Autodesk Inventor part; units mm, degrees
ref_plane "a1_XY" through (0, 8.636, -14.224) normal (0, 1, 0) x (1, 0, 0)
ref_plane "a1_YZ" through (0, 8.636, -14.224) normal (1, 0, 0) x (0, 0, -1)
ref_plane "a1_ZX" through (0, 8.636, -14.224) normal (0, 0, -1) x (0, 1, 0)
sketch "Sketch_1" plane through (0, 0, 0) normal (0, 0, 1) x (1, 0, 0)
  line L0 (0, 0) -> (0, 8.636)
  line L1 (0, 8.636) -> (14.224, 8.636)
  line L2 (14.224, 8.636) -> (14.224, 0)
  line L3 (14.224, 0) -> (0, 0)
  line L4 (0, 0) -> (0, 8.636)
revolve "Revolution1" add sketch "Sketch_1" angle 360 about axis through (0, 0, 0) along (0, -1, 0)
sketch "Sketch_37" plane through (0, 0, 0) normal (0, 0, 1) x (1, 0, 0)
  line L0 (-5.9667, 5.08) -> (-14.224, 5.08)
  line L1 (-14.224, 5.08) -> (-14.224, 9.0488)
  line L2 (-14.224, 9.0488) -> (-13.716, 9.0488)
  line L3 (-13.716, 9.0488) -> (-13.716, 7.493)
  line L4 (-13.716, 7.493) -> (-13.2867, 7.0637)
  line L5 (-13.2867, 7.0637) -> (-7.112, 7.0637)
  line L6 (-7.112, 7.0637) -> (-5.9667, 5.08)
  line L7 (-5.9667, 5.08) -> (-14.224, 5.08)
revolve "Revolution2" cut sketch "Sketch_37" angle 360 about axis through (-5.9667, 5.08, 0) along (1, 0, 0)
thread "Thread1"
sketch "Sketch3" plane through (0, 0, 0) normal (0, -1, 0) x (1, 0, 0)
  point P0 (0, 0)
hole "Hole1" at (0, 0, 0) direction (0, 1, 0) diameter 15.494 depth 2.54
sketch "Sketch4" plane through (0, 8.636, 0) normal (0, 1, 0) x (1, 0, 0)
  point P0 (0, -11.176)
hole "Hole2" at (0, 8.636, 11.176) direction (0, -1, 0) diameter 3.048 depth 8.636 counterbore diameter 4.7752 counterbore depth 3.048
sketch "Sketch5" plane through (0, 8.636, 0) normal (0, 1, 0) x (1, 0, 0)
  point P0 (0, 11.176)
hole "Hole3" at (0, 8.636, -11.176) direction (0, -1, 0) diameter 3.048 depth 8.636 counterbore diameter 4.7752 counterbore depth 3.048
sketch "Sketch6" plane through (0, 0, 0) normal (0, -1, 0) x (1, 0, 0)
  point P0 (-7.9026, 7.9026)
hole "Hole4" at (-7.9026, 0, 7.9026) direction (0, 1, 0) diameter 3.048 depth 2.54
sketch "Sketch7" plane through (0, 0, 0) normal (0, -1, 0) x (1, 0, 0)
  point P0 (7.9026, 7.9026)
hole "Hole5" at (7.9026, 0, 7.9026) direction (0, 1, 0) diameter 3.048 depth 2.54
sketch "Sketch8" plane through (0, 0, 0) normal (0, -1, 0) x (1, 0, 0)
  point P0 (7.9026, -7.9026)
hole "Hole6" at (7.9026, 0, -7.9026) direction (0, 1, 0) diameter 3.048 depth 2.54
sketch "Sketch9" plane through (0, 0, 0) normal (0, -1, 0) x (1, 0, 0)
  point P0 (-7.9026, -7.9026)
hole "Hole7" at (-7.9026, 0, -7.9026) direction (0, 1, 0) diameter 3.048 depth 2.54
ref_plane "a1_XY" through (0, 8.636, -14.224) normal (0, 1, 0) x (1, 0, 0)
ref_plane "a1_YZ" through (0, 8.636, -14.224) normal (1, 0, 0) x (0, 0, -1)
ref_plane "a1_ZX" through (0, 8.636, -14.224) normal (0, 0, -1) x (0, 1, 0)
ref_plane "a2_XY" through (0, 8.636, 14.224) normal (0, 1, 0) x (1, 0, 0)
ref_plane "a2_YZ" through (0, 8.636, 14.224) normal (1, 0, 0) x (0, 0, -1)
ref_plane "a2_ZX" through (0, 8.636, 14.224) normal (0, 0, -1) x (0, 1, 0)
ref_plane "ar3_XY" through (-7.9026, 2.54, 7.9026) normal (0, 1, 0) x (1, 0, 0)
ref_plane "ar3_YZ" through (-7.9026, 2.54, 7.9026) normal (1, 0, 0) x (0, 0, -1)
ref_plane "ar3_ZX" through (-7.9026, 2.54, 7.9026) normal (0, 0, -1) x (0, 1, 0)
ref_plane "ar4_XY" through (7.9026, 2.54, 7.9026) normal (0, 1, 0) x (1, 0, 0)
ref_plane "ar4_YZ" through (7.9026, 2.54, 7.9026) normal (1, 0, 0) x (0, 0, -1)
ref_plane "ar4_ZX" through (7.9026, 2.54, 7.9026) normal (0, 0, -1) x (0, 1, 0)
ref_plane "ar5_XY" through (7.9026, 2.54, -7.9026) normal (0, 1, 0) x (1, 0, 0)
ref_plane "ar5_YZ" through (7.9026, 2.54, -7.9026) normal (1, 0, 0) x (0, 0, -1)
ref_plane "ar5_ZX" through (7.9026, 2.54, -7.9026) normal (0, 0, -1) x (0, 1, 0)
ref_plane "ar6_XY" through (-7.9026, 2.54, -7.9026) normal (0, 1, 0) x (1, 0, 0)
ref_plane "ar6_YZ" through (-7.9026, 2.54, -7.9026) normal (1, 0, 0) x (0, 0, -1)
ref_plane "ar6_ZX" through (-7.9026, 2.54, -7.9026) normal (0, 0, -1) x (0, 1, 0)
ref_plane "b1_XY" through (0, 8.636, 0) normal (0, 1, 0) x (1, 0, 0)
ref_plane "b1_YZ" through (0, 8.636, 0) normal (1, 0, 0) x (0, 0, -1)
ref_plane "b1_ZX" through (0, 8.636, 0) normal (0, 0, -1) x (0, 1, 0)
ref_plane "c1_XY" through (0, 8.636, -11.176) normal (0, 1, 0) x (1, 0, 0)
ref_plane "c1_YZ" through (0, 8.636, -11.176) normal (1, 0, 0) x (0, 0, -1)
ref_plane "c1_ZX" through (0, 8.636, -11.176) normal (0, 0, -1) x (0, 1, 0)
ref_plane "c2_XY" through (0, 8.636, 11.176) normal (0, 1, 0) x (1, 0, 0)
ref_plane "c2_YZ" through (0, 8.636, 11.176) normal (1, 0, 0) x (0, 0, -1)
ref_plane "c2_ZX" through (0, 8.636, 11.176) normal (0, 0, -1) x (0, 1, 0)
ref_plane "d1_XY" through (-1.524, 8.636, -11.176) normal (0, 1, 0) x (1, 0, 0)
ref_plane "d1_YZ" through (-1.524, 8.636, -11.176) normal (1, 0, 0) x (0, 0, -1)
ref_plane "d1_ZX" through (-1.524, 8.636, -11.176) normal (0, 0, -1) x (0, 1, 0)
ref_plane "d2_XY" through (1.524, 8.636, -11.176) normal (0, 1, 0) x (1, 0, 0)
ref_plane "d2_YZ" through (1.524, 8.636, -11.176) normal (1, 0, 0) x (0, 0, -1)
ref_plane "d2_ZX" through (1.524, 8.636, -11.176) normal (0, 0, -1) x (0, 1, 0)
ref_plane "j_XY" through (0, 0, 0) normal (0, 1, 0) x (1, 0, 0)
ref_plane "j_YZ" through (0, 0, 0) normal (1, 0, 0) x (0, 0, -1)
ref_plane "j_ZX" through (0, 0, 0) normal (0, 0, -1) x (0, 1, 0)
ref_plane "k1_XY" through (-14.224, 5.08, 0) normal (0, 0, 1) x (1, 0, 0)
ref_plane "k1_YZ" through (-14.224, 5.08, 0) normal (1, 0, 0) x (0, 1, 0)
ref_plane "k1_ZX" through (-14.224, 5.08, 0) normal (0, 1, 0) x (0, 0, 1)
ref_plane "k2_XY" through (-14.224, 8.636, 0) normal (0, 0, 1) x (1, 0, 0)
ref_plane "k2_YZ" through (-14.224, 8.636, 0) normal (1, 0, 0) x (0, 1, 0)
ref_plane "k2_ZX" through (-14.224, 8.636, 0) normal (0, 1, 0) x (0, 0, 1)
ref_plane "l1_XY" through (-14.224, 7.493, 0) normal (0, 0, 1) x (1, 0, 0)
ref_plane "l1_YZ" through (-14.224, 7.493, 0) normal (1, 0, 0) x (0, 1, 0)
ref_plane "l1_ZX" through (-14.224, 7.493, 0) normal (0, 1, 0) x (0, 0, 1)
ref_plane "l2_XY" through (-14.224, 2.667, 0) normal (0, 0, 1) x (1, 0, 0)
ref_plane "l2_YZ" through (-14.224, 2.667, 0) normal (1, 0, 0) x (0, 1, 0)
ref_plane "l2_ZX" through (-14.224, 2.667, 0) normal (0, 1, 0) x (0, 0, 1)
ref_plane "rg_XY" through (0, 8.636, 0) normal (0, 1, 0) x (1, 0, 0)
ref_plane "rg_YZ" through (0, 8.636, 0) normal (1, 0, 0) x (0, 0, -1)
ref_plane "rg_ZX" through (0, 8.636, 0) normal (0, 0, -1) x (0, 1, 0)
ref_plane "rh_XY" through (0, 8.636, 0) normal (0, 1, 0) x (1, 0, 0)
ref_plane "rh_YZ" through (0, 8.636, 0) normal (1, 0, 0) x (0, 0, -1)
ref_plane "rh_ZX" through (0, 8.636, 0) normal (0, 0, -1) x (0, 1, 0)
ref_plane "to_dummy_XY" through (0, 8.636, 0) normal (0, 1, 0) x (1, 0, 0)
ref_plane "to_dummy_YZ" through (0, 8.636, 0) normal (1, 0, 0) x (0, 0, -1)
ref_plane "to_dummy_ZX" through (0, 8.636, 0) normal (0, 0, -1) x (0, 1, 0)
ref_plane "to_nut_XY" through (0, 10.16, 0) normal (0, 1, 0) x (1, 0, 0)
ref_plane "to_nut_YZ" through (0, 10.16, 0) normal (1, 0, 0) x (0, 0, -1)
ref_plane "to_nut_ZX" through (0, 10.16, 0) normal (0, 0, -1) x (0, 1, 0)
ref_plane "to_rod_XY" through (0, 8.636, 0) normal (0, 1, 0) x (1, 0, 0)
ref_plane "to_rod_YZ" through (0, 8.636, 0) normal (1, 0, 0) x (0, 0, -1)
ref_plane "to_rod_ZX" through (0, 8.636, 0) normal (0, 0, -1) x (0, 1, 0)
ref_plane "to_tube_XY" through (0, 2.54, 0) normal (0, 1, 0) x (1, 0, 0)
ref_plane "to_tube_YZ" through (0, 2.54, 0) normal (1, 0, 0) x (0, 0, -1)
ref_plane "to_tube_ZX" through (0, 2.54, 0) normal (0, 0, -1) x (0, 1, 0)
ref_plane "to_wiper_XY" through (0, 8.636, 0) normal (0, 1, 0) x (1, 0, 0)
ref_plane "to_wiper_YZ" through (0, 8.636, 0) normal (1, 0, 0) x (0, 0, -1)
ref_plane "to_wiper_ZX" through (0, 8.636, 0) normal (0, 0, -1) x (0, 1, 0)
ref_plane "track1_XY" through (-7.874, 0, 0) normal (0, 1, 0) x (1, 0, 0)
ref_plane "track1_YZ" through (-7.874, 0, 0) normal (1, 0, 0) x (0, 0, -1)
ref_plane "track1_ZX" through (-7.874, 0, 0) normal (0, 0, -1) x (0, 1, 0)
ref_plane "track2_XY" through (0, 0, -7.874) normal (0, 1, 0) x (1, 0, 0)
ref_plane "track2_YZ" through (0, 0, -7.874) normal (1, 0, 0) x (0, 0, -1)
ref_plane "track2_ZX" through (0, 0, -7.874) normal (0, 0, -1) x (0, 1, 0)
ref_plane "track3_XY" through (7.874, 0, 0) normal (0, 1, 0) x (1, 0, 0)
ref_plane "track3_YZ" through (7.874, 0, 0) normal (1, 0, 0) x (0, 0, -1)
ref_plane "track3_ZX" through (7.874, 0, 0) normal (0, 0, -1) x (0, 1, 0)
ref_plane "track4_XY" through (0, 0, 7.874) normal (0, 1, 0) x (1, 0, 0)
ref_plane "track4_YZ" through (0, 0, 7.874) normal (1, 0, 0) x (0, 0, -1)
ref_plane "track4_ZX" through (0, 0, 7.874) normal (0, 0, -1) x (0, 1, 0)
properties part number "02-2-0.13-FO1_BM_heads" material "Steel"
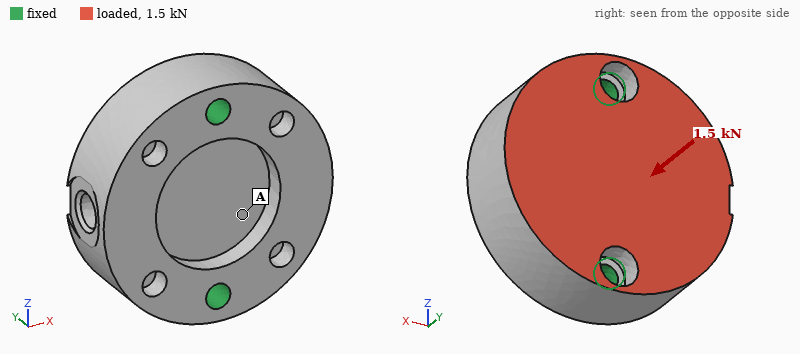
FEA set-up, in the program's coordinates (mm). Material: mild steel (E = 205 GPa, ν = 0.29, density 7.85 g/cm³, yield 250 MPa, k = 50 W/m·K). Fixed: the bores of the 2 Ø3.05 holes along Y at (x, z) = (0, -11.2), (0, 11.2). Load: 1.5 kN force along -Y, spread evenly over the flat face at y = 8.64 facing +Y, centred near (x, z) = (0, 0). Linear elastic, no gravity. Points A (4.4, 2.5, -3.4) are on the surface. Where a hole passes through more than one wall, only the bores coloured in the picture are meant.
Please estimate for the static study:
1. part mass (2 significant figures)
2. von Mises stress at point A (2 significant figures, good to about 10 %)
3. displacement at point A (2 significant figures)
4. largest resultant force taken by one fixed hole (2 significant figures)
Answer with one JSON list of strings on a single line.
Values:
["36 g", "7.5 MPa", "1.3 µm", "810 N"]
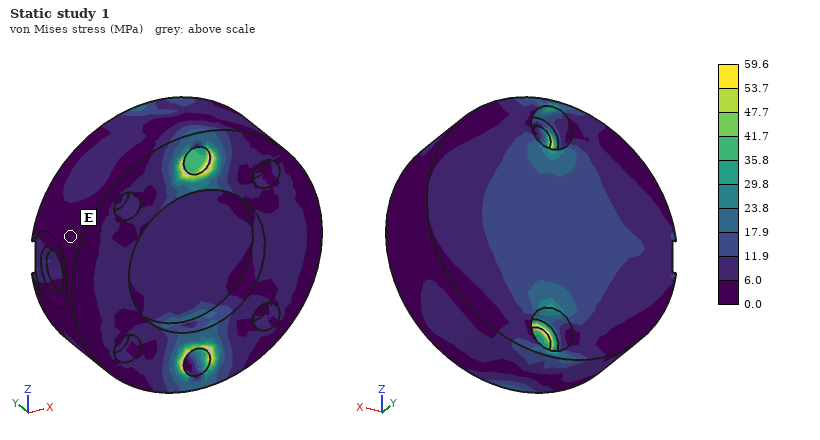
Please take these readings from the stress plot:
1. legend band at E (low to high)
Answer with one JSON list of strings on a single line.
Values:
["0.0 to 6.0 MPa"]
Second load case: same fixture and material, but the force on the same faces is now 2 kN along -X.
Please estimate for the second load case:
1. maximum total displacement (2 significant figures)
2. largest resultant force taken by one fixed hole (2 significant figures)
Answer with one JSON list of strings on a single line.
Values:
["7.5 µm", "1.0 kN"]
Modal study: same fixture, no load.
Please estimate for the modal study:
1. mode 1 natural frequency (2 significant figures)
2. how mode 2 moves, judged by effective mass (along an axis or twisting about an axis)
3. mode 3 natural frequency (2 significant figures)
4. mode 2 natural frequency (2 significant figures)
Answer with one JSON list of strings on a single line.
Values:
["17 kHz", "along Y", "42 kHz", "26 kHz"]
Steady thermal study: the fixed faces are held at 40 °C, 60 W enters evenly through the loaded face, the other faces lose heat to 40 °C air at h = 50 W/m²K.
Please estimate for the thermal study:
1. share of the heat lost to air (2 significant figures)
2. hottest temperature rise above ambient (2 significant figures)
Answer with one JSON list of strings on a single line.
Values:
["4.6 %", "52 K"]
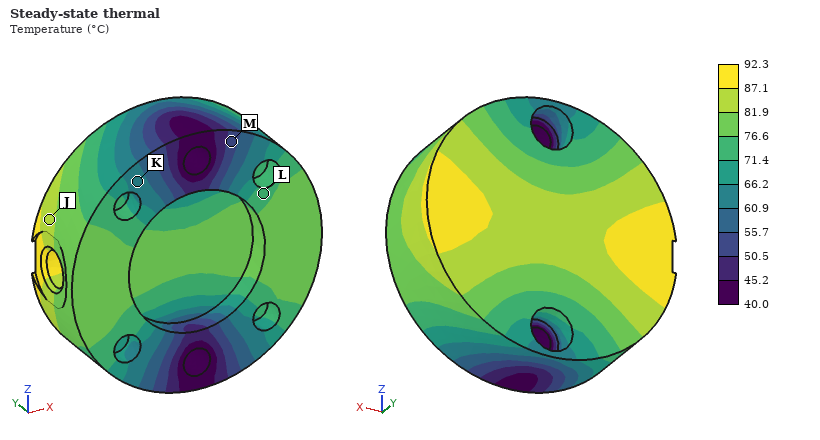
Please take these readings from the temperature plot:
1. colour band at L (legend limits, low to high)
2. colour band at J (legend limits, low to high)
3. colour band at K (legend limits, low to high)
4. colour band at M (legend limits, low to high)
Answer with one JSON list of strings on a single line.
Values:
["71.4 to 76.6 °C", "81.9 to 87.1 °C", "60.9 to 66.2 °C", "50.5 to 55.7 °C"]
